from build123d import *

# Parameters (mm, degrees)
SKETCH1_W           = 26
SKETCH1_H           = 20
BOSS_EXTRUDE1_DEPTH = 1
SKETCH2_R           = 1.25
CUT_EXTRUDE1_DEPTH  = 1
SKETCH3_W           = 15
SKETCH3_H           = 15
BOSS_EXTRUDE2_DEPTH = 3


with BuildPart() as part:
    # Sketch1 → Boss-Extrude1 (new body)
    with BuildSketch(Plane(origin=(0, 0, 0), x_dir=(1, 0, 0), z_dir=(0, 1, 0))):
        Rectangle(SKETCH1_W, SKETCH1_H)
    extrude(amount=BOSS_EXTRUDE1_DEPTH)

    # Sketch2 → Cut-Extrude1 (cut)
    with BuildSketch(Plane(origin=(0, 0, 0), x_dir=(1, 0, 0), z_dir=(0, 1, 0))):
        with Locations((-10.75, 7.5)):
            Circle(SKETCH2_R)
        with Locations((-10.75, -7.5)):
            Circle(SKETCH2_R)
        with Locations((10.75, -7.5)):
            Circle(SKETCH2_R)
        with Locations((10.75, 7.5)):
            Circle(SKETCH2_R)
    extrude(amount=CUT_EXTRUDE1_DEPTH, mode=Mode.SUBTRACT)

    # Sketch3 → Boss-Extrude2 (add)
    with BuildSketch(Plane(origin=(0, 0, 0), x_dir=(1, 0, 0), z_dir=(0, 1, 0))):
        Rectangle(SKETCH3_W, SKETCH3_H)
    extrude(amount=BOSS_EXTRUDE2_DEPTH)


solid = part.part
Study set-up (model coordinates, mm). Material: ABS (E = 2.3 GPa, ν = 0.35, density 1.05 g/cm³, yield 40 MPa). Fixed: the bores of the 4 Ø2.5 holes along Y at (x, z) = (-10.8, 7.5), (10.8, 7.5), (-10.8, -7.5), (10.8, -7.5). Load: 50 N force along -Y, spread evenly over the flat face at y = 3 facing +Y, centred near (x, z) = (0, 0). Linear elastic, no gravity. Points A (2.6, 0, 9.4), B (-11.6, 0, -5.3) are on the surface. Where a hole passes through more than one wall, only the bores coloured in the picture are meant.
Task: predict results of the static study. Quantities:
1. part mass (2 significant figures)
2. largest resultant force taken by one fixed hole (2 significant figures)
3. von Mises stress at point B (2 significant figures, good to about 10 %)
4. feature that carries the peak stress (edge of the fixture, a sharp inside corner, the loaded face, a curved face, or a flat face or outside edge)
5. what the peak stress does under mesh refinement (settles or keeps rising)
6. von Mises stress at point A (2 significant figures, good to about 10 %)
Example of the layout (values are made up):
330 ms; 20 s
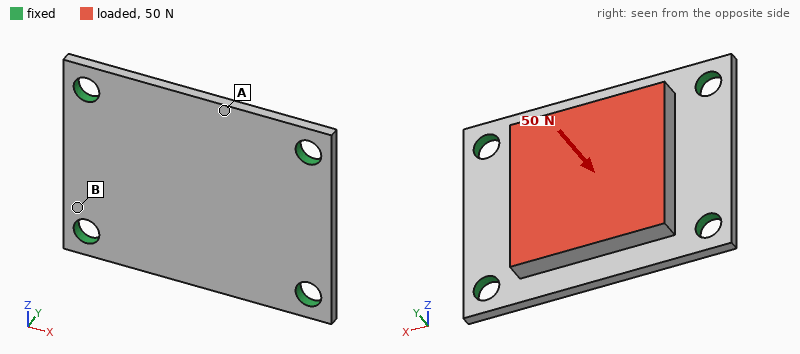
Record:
1.00 g; 18 N; 5.2 MPa; edge of the fixture; keeps rising; 2.4 MPa
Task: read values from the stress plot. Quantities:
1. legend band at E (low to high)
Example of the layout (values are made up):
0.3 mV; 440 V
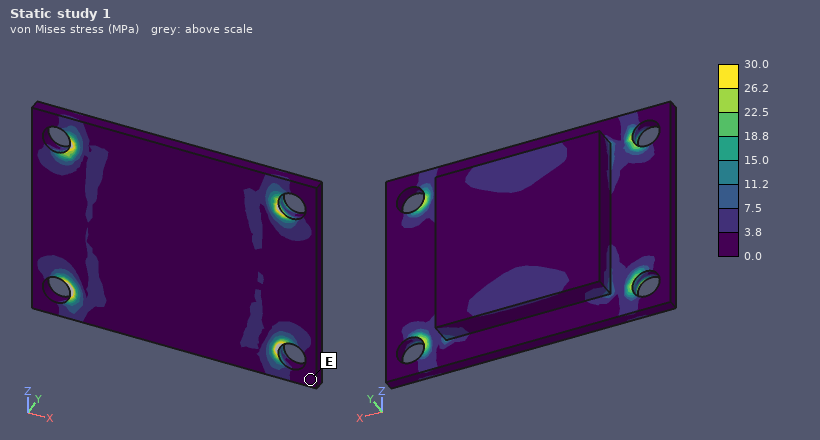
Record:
0.0 to 3.8 MPa
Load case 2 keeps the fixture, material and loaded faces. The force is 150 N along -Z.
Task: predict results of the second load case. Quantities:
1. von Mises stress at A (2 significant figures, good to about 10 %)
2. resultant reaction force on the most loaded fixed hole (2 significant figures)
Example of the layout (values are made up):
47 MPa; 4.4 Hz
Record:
4.0 MPa; 47 N
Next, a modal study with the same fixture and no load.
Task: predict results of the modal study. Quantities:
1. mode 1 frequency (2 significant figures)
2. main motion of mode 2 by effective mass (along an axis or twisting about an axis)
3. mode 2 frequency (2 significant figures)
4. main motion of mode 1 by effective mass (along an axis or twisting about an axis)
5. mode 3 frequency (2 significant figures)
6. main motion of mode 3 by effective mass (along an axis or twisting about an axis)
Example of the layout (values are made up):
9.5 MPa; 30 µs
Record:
4900 Hz; twisting about X; 6900 Hz; along Y; 9400 Hz; twisting about Z
